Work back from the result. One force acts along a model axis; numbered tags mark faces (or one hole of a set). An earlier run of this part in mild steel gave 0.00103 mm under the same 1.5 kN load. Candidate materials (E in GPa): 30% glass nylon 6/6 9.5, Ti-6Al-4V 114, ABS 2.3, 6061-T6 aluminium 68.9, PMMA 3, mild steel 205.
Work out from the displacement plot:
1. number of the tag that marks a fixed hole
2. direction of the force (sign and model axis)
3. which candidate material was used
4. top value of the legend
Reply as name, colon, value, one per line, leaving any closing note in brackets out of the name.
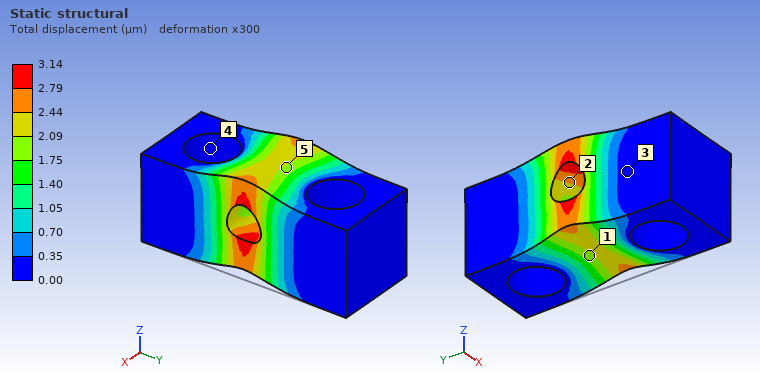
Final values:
number of the tag that marks a fixed hole: 4
direction of the force: +Z
which candidate material was used: 6061-T6 aluminium
top value of the legend: 3.14 µm
